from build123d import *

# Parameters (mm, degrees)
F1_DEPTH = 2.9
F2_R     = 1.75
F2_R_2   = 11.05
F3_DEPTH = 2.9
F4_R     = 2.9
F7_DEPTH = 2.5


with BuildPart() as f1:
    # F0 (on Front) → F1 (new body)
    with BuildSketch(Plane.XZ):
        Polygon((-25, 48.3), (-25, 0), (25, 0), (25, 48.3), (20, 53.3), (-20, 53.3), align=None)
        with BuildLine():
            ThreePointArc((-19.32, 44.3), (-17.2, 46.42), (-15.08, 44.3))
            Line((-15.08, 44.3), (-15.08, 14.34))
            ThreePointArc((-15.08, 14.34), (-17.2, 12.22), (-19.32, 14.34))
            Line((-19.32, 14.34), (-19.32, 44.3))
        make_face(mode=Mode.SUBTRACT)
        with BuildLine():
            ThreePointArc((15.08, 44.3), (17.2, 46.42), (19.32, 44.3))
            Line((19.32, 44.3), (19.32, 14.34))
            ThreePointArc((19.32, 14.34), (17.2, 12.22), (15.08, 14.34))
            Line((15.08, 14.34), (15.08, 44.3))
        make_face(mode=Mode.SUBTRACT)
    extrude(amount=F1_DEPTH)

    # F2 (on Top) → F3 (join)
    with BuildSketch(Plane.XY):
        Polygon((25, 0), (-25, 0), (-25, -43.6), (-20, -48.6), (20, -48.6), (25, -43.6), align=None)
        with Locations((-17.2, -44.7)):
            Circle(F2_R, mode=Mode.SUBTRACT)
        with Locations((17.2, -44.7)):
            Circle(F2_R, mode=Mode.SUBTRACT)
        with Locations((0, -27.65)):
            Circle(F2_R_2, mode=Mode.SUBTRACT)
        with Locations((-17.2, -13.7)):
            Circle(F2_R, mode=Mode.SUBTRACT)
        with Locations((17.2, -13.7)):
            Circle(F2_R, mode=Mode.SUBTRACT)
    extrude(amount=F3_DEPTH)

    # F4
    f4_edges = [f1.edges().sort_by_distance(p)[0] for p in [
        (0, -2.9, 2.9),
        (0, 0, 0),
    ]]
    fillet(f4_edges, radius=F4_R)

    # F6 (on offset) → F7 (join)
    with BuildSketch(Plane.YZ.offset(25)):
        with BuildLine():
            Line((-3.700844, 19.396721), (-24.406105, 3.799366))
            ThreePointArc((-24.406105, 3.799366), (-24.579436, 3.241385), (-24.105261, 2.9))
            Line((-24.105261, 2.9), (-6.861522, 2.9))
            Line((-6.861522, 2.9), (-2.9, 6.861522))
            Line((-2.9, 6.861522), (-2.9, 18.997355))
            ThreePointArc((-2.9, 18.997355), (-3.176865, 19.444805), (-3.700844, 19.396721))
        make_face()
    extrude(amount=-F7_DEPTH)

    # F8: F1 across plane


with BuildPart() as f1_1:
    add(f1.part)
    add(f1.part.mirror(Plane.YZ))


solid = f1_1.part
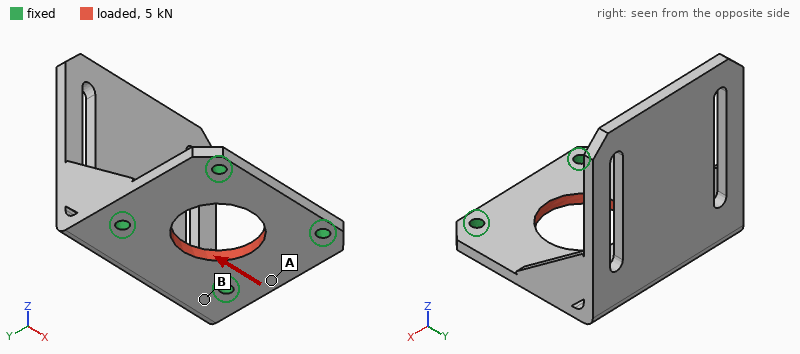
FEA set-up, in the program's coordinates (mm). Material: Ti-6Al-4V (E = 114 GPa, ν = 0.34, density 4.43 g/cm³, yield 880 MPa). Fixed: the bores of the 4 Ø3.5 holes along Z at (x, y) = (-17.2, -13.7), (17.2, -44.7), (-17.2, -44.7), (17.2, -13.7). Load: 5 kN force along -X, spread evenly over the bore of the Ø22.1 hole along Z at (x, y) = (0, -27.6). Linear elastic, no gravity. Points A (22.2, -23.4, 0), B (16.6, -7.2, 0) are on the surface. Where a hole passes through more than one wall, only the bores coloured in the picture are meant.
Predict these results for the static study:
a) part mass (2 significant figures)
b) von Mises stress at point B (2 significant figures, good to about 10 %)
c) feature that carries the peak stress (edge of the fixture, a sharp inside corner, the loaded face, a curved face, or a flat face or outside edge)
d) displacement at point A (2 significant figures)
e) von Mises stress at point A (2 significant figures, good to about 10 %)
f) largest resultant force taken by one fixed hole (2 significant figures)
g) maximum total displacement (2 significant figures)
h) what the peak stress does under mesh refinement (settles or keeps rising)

58 g
8.0 MPa
edge of the fixture
4.8 µm
21 MPa
1.4 kN
7.3 µm
keeps rising
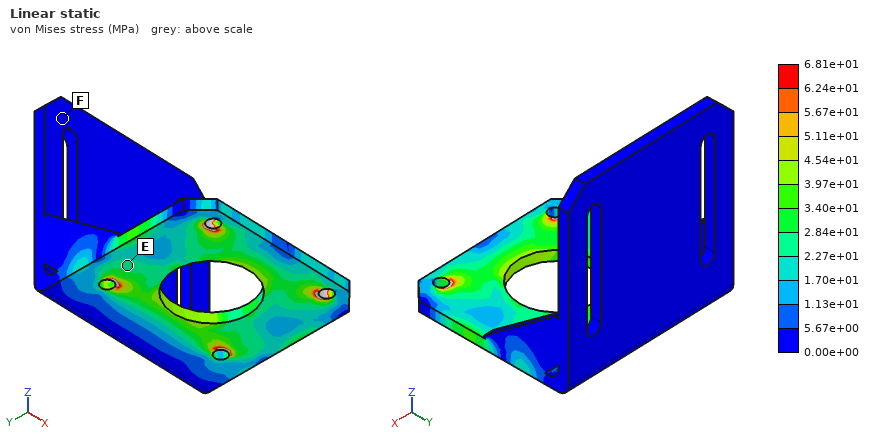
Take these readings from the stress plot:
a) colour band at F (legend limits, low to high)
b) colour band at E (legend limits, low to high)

0.00e+00 to 5.67e+00 MPa
2.27e+01 to 2.84e+01 MPa
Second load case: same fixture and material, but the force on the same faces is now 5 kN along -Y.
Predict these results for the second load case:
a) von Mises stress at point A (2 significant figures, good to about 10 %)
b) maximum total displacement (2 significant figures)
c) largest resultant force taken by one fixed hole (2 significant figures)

7.8 MPa
11 µm
1.4 kN
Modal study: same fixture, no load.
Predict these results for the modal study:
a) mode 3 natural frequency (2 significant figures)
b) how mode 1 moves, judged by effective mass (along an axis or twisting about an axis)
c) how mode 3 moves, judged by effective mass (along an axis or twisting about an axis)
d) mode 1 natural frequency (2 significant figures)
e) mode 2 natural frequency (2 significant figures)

3600 Hz
along Y
along X
1000 Hz
2400 Hz
